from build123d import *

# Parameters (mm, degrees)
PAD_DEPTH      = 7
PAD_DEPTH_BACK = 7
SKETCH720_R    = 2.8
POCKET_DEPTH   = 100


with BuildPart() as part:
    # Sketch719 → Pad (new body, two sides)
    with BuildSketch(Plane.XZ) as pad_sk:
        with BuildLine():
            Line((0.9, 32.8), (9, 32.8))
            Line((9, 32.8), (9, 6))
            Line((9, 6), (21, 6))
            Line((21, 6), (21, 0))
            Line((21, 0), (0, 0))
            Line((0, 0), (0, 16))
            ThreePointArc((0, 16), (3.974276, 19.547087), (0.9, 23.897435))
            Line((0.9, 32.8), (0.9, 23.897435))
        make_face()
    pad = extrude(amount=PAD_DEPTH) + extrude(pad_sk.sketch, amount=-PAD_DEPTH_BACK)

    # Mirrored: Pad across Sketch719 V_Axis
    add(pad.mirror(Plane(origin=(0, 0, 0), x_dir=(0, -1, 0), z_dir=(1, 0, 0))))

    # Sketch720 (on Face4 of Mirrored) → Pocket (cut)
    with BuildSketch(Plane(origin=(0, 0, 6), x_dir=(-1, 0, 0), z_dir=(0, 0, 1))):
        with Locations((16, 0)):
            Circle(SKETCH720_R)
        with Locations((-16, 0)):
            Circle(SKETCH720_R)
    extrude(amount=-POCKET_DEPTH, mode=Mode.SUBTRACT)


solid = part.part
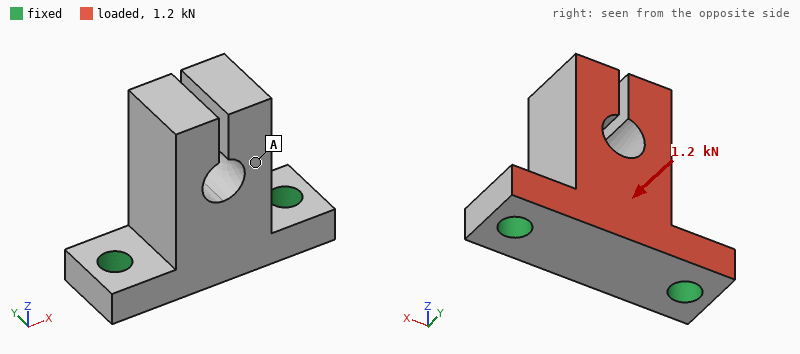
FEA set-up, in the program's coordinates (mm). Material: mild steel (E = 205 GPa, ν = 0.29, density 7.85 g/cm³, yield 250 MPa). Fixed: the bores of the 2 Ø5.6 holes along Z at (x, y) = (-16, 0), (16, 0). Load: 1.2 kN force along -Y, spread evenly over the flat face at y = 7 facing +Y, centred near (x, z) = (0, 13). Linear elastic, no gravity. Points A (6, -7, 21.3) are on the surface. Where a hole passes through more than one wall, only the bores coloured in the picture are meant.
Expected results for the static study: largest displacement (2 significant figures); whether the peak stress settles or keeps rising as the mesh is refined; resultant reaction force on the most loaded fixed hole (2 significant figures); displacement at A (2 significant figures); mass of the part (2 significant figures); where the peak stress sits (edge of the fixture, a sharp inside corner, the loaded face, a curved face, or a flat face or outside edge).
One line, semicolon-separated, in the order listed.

23 µm; keeps rising; 600 N; 15 µm; 71 g; edge of the fixture
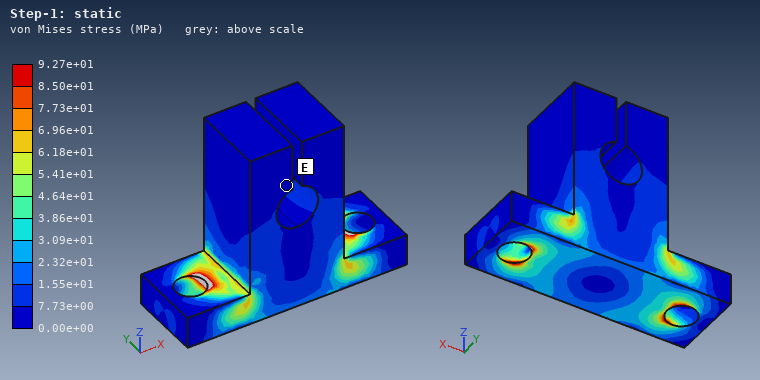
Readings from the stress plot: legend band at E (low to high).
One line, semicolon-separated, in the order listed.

0.00e+00 to 7.73e+00 MPa
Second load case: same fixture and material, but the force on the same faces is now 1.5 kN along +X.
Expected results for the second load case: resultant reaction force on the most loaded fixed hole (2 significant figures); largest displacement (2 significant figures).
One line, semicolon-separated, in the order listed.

1.0 kN; 15 µm
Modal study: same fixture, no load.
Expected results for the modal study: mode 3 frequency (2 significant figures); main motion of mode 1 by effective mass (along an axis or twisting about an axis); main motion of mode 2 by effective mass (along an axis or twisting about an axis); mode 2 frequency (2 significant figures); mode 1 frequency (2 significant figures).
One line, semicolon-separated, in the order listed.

9900 Hz; along Y; along X; 8100 Hz; 5100 Hz
